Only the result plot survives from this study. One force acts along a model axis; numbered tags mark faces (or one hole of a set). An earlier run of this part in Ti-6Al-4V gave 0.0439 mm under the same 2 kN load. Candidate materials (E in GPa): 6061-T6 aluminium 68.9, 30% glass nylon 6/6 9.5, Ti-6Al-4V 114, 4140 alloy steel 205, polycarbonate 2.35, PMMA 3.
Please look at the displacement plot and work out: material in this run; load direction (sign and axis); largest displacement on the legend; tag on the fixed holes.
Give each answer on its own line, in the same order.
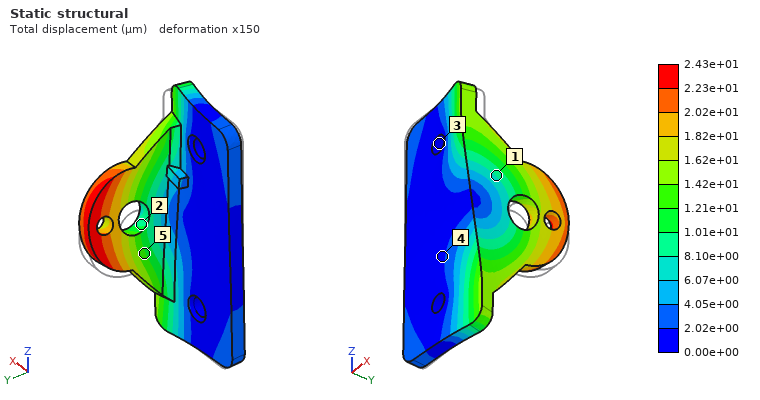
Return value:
4140 alloy steel
+Z
2.43e+01 µm
3
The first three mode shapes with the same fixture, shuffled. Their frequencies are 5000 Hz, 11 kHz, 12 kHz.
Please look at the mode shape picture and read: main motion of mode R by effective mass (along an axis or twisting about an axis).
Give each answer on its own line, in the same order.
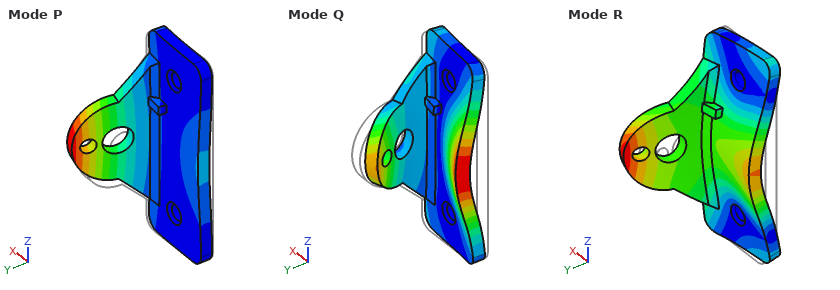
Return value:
along Y
